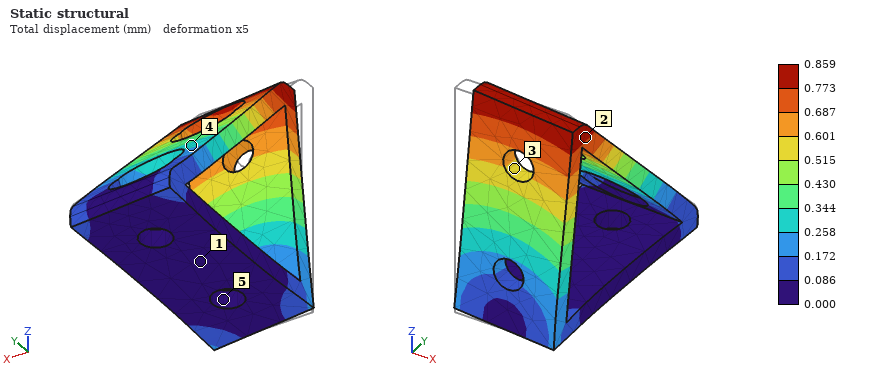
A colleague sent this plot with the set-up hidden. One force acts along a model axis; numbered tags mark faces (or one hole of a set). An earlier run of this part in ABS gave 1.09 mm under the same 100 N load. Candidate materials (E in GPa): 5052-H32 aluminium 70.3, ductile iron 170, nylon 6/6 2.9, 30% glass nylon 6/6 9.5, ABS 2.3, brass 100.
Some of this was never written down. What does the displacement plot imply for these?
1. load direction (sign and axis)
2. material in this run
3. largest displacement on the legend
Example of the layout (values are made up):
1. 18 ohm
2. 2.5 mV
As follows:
1. +X
2. nylon 6/6
3. 0.859 mm
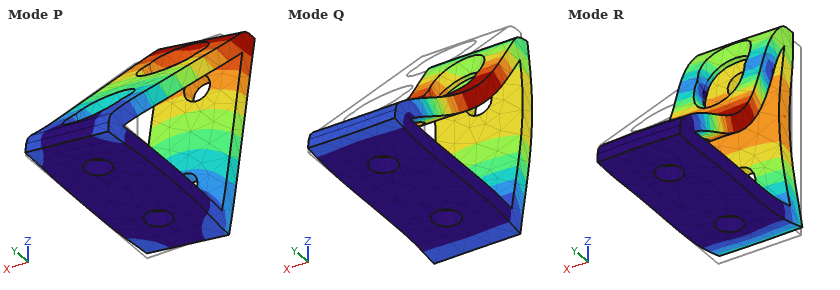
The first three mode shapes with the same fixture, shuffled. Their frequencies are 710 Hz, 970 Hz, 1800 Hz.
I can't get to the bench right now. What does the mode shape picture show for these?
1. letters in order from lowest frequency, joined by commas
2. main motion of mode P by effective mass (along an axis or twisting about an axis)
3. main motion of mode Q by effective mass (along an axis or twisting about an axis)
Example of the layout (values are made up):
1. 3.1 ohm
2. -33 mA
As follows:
1. P, Q, R
2. along X
3. along Y
